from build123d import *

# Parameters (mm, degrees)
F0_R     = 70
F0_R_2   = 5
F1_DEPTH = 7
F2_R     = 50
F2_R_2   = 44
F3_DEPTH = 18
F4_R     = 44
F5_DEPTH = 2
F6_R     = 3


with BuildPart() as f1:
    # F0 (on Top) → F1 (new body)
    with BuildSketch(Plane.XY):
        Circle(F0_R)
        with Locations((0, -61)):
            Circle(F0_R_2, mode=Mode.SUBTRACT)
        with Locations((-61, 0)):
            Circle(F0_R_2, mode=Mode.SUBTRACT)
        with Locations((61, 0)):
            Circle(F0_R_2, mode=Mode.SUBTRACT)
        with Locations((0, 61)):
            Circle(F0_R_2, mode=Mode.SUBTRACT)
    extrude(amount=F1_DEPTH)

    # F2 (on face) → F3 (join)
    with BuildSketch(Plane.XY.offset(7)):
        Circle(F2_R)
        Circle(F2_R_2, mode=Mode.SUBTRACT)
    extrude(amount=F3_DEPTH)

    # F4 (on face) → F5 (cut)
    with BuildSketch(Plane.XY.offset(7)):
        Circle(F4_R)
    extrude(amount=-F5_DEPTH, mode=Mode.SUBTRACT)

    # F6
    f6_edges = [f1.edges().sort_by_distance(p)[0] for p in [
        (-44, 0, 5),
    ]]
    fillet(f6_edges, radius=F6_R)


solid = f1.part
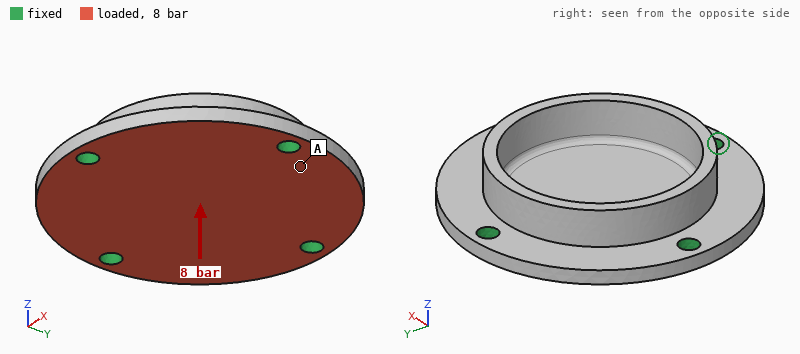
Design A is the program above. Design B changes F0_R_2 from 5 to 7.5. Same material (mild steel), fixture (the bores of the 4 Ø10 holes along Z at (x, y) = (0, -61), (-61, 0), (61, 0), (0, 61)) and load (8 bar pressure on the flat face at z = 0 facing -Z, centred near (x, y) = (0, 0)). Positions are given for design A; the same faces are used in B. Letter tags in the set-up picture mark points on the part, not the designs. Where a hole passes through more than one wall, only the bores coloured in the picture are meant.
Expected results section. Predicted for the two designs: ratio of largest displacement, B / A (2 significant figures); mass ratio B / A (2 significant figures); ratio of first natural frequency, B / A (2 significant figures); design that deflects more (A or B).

0.89
0.98
1.1
A
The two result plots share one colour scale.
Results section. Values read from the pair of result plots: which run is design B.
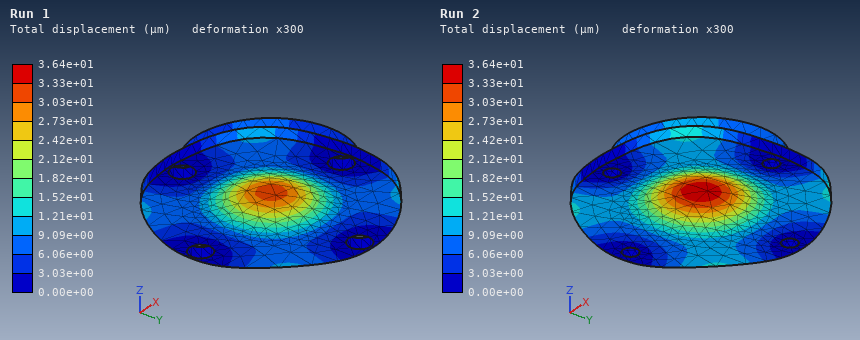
Run 1
